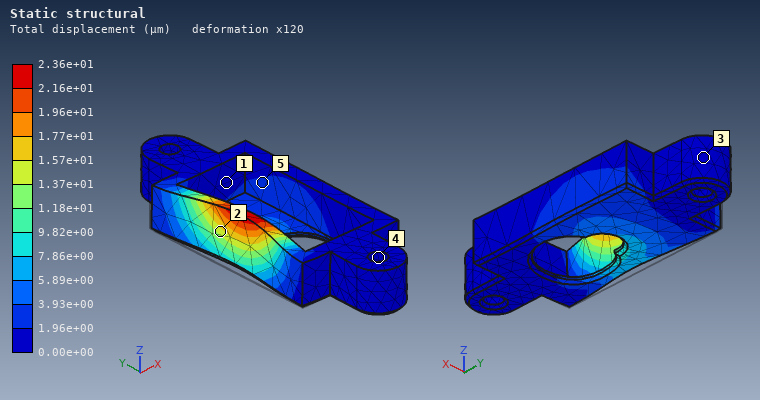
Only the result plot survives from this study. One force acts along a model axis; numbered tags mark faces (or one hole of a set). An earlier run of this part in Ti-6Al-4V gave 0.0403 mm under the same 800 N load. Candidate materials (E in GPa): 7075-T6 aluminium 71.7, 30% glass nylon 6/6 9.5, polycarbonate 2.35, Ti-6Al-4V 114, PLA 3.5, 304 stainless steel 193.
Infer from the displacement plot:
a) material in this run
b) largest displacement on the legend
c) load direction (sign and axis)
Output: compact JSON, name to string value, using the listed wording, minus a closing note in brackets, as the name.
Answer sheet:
{"material in this run": "304 stainless steel", "largest displacement on the legend": "2.36e+01 µm", "load direction": "+X"}
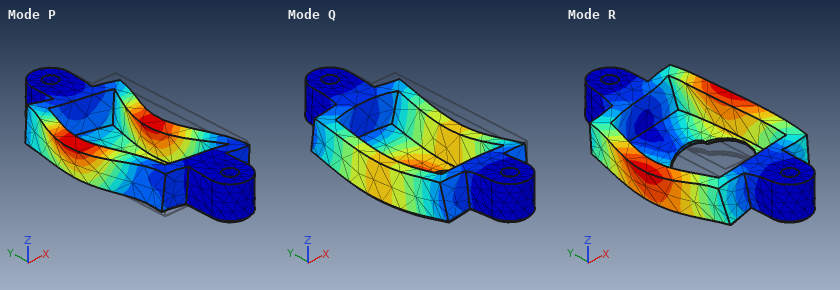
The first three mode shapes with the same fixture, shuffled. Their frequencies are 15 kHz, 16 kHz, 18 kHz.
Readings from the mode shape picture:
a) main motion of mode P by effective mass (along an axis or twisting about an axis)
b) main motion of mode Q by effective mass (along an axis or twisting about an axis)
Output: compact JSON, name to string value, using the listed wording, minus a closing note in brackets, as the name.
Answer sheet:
{"main motion of mode P by effective mass": "along X", "main motion of mode Q by effective mass": "along Z"}
